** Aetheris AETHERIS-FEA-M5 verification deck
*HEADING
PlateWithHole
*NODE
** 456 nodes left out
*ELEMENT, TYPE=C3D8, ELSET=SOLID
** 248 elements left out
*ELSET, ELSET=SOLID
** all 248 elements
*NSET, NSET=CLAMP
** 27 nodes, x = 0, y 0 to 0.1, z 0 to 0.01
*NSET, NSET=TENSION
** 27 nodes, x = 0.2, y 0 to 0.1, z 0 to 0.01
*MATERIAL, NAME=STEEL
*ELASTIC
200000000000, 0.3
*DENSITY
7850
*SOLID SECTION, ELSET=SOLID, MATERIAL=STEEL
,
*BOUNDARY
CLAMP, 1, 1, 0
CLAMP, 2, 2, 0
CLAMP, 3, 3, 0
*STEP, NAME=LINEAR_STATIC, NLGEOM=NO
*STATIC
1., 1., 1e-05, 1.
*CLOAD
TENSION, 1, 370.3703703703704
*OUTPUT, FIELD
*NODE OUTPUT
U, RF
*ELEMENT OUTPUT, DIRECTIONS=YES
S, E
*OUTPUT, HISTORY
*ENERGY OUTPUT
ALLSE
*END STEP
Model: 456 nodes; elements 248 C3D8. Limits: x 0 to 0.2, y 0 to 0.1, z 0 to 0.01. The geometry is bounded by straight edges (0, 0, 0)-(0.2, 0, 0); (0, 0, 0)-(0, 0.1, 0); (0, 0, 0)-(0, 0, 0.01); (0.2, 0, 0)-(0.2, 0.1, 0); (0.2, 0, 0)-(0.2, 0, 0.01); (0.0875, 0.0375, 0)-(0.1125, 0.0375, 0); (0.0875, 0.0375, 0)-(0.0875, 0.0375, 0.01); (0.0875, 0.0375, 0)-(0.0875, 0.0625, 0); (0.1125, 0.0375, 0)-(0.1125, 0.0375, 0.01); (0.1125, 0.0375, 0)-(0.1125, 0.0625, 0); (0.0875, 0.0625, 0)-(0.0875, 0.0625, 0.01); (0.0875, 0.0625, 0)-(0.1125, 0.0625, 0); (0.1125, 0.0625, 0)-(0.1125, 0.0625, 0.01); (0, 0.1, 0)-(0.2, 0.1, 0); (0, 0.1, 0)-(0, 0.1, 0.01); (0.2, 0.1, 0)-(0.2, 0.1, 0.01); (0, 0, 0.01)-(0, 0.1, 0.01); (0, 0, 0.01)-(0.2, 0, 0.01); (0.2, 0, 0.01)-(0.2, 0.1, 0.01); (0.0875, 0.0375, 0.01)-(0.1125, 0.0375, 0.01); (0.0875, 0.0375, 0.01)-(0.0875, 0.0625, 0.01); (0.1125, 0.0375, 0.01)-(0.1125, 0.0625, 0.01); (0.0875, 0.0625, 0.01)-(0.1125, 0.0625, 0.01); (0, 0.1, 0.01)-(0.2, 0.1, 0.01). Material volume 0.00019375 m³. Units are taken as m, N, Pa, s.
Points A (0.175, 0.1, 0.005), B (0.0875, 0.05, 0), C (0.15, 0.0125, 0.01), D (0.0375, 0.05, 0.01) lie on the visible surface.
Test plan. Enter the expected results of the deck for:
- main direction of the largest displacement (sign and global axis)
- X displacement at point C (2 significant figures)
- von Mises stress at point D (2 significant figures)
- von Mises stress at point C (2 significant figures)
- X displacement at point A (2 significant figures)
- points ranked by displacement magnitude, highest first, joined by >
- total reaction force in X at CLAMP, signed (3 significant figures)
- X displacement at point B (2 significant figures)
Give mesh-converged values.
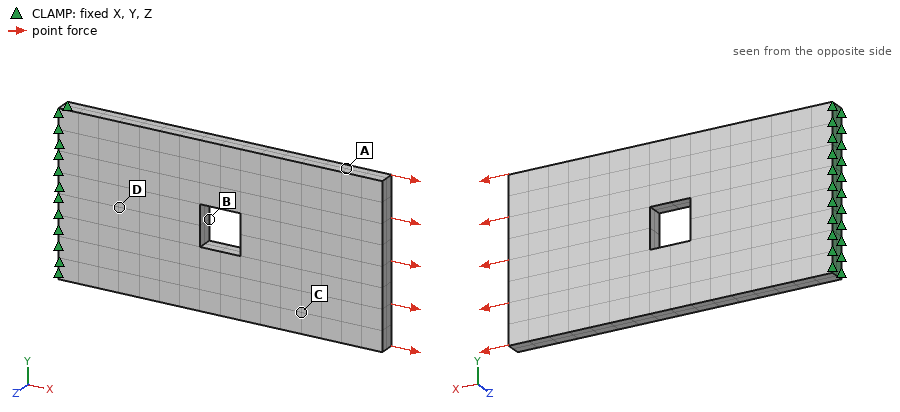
+X
8.4e-06 m
8.7e+06 Pa
1.1e+07 Pa
9.9e-06 m
A > C > B > D
-10000 N
3.1e-06 m
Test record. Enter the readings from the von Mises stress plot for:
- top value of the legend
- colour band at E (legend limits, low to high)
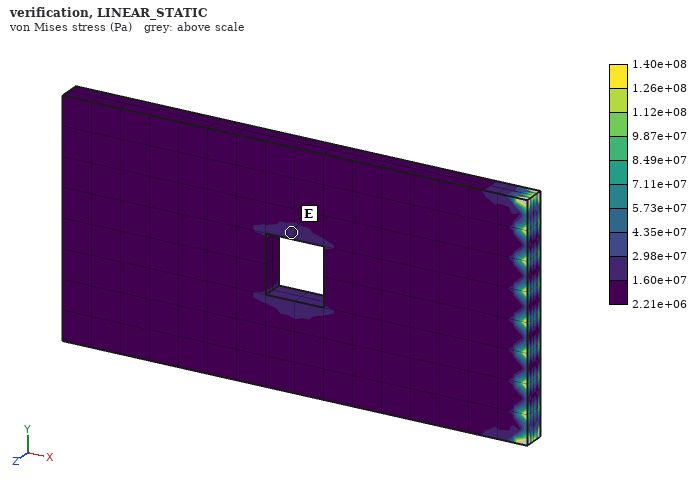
1.40e+08 Pa
1.60e+07 to 2.98e+07 Pa
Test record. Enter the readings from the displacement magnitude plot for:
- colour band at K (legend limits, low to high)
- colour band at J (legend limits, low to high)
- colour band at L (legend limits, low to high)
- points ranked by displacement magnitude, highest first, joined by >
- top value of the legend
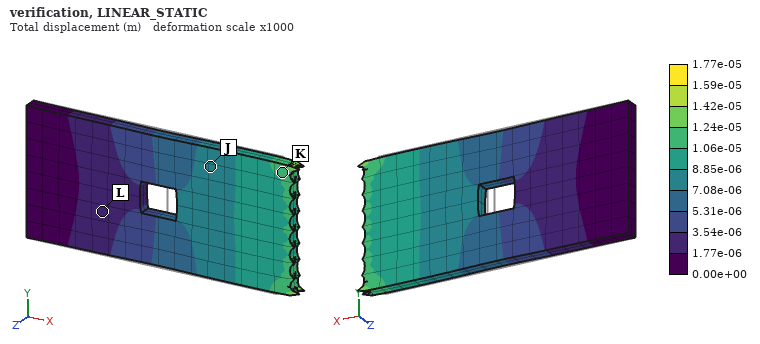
1.06e-05 to 1.24e-05 m
7.08e-06 to 8.85e-06 m
1.77e-06 to 3.54e-06 m
K > J > L
1.77e-05 m
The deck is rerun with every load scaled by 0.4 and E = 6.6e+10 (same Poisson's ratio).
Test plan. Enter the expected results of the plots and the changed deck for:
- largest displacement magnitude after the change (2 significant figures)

2.1e-05 m
